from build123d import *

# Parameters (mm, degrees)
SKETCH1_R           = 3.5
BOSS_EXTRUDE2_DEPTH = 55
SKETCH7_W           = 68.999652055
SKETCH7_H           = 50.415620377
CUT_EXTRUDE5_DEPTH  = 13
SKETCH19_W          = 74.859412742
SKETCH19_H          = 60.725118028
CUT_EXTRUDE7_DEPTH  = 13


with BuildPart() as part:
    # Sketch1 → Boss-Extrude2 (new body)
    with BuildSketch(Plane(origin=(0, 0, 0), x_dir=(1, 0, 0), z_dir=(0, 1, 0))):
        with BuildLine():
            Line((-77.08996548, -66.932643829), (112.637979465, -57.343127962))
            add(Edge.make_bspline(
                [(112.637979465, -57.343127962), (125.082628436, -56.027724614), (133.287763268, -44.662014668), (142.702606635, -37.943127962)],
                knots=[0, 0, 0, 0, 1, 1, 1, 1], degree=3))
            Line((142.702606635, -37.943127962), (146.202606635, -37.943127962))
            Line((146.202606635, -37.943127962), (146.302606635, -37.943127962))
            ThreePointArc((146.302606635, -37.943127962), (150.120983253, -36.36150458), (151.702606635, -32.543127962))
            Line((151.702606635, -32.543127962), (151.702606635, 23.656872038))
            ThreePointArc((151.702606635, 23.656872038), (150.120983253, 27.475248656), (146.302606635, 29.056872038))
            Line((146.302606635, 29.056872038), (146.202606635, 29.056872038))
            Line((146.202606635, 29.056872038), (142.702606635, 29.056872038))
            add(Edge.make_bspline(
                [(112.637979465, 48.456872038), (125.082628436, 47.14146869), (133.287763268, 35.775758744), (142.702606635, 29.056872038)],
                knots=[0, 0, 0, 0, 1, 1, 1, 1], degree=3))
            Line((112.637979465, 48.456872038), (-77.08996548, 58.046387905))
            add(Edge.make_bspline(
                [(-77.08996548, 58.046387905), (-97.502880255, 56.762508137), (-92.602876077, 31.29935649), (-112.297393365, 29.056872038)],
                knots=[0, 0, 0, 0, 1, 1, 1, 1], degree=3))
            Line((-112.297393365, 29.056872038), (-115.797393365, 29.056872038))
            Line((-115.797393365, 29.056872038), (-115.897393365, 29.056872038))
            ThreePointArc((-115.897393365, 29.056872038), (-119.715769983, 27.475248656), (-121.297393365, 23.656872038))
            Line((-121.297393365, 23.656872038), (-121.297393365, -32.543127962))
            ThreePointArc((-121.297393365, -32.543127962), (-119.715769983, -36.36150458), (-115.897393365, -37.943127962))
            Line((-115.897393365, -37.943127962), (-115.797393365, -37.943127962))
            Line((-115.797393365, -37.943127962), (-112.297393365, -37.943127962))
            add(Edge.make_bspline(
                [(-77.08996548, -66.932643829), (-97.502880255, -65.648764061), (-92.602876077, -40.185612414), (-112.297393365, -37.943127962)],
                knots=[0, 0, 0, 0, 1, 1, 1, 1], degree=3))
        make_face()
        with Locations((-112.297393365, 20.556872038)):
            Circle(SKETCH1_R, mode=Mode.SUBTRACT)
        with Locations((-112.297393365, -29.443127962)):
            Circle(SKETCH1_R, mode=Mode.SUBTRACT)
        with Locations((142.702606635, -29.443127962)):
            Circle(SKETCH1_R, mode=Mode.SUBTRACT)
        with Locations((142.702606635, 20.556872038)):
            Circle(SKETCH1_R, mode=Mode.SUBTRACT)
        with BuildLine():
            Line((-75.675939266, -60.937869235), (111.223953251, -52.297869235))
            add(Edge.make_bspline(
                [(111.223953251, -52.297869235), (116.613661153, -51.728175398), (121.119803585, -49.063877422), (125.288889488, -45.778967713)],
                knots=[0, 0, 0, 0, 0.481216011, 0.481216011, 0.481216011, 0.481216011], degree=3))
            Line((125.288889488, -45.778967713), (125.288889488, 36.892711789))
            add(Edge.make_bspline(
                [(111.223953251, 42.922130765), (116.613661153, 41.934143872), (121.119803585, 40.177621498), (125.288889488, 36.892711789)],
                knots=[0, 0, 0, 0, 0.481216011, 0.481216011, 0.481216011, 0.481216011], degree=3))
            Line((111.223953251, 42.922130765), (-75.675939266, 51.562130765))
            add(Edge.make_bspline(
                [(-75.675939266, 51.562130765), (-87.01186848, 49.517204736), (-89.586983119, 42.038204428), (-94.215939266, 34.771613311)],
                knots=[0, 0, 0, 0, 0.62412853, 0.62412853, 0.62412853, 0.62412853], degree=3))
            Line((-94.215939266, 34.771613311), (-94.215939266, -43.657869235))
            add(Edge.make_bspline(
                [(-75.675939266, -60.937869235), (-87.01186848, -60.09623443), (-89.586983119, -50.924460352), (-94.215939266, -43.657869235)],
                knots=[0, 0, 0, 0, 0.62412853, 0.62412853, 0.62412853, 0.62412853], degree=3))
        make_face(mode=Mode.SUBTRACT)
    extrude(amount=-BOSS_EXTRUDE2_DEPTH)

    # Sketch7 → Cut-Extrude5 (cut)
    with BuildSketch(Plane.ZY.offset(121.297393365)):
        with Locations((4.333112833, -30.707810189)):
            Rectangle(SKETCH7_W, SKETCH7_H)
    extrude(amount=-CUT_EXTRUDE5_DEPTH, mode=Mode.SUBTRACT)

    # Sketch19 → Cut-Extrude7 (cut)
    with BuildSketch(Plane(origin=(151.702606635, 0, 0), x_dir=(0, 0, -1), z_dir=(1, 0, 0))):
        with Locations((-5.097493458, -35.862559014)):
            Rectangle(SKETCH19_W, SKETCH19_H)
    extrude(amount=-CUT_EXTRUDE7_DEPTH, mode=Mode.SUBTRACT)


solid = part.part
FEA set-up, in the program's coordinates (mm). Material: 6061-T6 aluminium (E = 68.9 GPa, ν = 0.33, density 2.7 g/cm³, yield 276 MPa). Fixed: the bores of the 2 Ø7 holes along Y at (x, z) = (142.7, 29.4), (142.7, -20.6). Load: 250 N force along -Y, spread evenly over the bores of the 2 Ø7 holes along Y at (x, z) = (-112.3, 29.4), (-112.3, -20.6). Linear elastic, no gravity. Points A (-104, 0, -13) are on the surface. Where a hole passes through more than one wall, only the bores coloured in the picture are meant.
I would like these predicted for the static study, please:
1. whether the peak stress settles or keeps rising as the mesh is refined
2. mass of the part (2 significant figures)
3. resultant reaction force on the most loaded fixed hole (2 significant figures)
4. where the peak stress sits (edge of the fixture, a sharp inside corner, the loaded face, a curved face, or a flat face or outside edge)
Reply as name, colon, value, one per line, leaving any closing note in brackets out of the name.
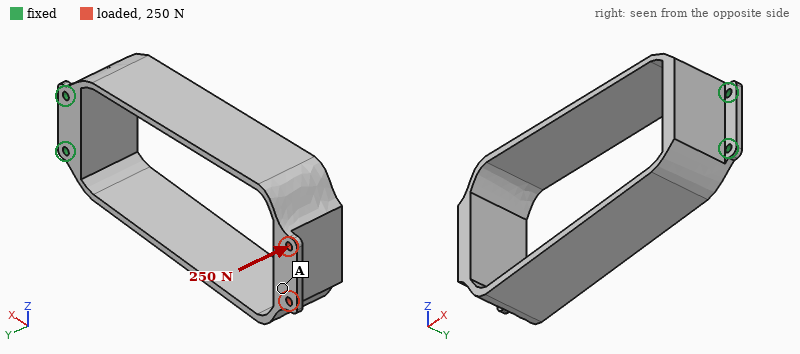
whether the peak stress settles or keeps rising as the mesh is refined: keeps rising
mass of the part: 750 g
resultant reaction force on the most loaded fixed hole: 610 N
where the peak stress sits: edge of the fixture
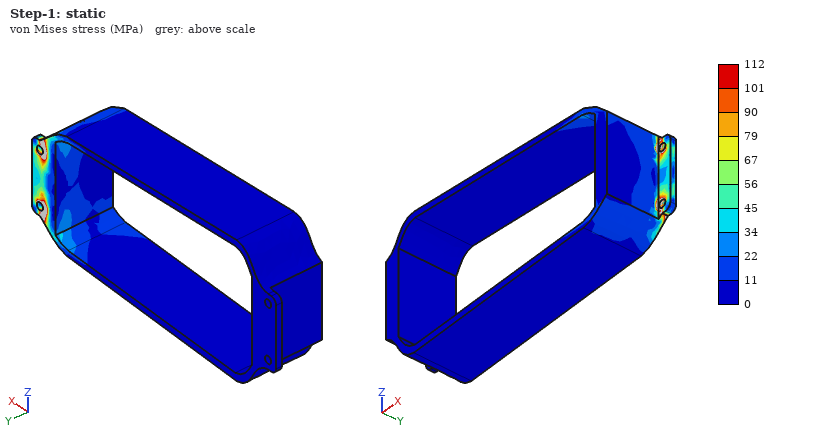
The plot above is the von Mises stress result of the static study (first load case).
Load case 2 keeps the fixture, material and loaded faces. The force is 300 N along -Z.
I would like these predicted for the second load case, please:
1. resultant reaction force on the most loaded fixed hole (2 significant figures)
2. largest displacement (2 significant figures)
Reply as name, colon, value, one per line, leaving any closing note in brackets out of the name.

resultant reaction force on the most loaded fixed hole: 1.4 kN
largest displacement: 3.6 mm
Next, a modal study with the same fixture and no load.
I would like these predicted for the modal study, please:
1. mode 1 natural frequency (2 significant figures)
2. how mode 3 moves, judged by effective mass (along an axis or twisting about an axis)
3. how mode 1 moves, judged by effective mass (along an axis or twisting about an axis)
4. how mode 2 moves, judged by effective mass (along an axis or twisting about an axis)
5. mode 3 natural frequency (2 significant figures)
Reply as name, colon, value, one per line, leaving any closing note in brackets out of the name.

mode 1 natural frequency: 83 Hz
how mode 3 moves, judged by effective mass: twisting about X
how mode 1 moves, judged by effective mass: along Z
how mode 2 moves, judged by effective mass: along Y
mode 3 natural frequency: 380 Hz
